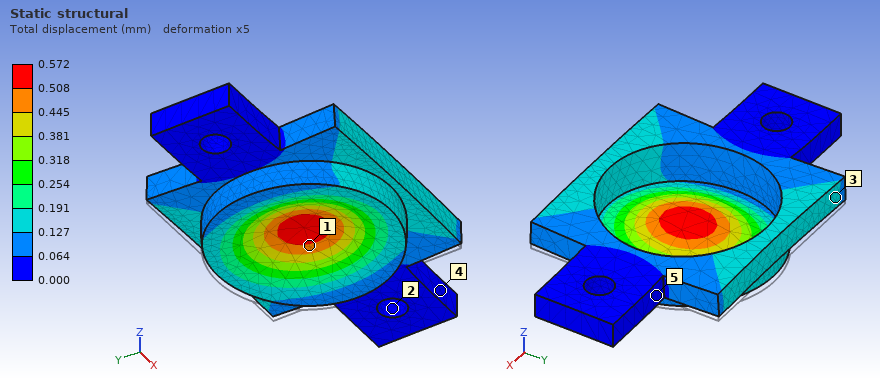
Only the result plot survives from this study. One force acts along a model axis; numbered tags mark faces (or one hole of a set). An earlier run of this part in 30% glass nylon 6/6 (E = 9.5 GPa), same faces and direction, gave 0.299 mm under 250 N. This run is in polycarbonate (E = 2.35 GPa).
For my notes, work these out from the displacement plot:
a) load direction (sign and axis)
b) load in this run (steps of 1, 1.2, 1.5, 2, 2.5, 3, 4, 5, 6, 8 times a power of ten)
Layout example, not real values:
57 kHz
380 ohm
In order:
+Z
120 N
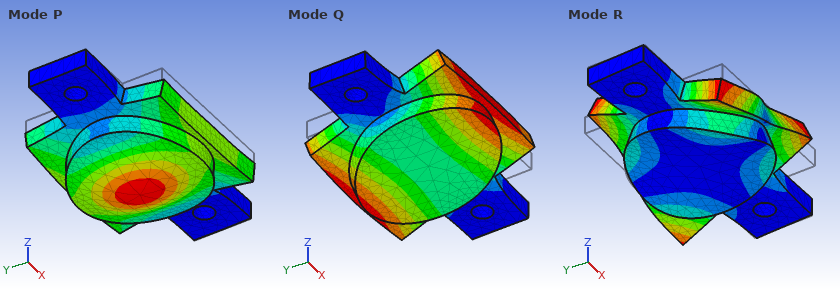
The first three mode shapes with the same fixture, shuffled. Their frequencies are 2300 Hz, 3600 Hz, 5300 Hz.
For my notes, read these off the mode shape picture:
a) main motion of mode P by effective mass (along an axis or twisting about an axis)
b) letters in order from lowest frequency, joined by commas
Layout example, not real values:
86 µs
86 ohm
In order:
along Z
Q, P, R
